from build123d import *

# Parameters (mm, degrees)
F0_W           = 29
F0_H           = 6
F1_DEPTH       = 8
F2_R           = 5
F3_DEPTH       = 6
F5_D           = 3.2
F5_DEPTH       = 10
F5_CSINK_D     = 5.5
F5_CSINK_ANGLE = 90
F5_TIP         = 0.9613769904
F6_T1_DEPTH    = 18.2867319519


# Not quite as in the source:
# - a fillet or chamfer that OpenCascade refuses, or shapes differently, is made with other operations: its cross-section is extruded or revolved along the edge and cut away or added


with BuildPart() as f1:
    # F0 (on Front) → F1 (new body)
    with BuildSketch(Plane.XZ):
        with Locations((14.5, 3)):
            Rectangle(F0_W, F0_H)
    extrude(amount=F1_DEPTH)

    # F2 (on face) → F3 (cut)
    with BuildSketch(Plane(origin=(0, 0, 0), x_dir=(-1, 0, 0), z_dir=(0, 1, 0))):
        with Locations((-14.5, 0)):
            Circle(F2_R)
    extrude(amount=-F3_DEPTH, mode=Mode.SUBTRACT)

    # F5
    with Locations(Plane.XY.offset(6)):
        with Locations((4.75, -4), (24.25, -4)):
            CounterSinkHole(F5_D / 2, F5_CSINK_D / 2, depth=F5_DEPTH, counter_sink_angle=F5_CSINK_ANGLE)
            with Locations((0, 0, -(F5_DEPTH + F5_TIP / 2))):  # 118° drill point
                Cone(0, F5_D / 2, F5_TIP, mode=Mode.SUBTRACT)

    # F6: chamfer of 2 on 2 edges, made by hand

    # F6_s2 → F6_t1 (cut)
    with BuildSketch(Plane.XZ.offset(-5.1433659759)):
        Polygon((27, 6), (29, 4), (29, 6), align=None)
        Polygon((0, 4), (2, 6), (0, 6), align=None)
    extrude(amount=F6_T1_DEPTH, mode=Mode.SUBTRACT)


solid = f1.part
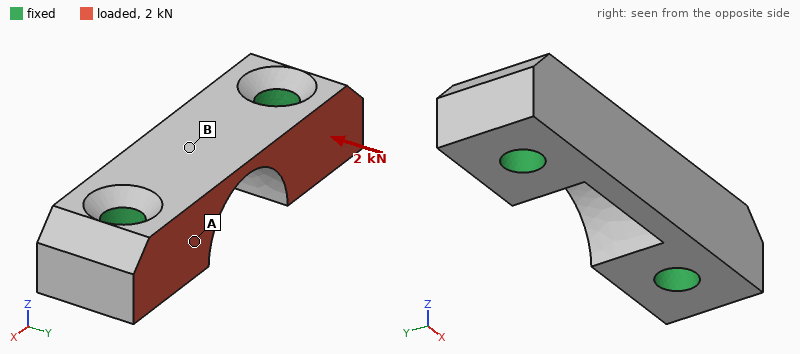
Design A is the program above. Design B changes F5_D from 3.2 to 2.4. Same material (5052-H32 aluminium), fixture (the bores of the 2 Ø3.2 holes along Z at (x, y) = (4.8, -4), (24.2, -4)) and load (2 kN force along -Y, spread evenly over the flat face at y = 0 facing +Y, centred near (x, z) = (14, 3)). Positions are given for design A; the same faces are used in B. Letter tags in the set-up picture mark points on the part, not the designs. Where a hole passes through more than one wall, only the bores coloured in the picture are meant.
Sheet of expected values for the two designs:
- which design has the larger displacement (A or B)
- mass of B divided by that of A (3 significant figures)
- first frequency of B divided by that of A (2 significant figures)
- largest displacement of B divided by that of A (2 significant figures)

B
1.03
0.83
1.3
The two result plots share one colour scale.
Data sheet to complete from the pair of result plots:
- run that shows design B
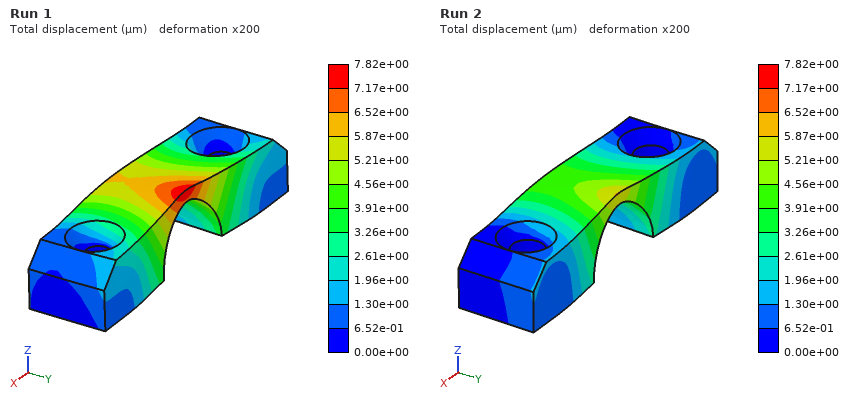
Run 1
